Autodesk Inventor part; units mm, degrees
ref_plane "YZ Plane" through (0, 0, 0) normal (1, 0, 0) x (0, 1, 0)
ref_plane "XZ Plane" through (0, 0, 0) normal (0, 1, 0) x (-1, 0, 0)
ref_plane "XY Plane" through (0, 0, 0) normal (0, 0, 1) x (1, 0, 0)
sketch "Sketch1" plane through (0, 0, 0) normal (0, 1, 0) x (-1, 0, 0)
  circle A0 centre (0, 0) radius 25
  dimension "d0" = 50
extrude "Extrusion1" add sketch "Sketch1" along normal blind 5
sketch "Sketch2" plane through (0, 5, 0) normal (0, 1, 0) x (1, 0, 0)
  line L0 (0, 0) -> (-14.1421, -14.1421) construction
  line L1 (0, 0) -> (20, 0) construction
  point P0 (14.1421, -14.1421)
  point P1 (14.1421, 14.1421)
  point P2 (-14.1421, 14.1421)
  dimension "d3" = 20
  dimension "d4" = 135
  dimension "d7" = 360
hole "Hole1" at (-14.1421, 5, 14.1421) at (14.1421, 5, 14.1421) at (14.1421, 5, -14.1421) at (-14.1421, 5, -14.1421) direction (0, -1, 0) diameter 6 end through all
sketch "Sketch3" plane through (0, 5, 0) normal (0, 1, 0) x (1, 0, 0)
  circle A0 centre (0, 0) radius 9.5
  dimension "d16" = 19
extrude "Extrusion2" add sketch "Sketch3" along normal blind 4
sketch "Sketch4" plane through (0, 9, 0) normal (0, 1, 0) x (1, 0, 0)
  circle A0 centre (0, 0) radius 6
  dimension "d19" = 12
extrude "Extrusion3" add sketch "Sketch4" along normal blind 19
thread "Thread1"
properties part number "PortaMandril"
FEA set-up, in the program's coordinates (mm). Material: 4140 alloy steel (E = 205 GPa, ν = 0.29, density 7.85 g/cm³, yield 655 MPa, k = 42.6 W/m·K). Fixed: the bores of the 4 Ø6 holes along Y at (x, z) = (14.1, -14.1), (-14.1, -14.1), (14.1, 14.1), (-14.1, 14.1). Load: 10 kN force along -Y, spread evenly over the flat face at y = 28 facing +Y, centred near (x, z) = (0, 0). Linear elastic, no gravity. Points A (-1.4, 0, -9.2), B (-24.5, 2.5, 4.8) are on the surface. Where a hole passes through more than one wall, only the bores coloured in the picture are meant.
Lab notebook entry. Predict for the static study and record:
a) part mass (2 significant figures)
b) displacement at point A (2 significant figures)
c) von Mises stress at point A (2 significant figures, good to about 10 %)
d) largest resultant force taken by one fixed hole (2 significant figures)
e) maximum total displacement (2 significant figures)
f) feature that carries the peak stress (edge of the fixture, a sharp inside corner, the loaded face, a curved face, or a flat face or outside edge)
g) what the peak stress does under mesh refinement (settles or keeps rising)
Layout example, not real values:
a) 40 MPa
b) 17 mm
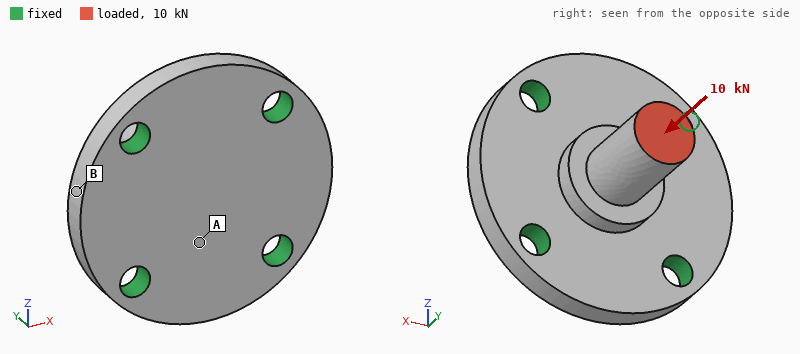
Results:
a) 98 g
b) 13 µm
c) 85 MPa
d) 2.6 kN
e) 24 µm
f) edge of the fixture
g) keeps rising
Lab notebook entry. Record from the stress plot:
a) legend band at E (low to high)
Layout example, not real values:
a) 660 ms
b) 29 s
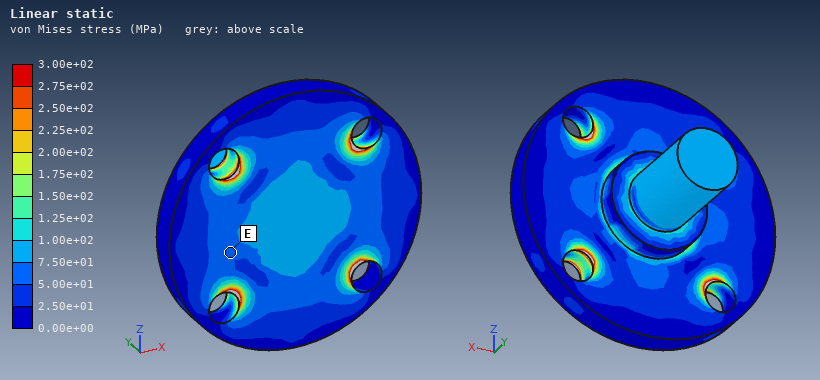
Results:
a) 5.00e+01 to 7.50e+01 MPa
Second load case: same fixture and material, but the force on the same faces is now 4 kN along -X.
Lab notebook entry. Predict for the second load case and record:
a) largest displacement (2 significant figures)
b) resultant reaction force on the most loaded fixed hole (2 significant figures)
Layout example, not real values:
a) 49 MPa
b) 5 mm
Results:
a) 0.11 mm
b) 2.4 kN
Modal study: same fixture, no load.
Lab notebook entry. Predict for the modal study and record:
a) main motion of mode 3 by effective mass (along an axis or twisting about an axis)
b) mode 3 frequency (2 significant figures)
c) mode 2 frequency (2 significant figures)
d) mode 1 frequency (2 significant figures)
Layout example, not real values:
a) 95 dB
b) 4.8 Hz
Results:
a) along Y
b) 19 kHz
c) 13 kHz
d) 13 kHz
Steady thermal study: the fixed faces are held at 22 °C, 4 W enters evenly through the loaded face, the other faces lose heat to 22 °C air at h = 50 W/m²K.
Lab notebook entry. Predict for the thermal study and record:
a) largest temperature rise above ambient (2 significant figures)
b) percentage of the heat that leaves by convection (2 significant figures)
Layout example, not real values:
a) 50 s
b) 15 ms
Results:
a) 20 K
b) 17 %
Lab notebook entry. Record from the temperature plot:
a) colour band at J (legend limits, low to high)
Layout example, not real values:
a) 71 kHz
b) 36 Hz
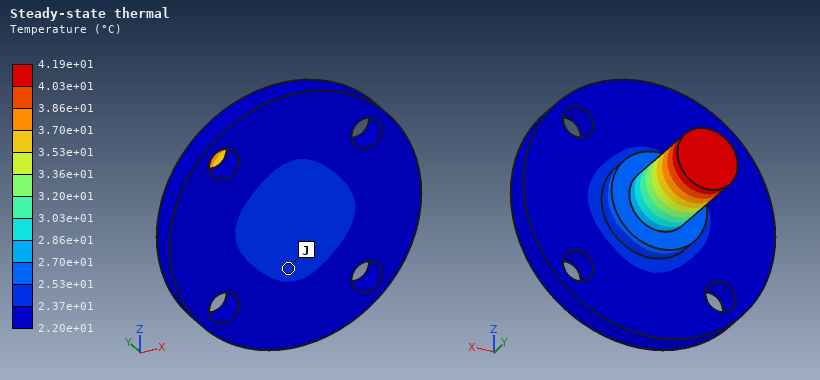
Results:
a) 2.37e+01 to 2.53e+01 °C
